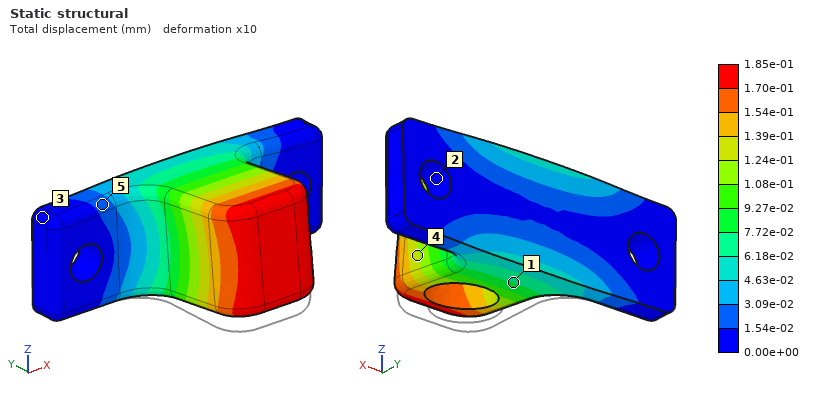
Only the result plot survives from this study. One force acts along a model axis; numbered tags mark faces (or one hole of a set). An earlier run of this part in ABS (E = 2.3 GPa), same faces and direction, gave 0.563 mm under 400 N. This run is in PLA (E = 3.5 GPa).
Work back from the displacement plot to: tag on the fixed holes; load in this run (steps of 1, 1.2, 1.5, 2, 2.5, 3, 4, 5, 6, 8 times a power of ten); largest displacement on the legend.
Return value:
2
200 N
1.85e-01 mm
